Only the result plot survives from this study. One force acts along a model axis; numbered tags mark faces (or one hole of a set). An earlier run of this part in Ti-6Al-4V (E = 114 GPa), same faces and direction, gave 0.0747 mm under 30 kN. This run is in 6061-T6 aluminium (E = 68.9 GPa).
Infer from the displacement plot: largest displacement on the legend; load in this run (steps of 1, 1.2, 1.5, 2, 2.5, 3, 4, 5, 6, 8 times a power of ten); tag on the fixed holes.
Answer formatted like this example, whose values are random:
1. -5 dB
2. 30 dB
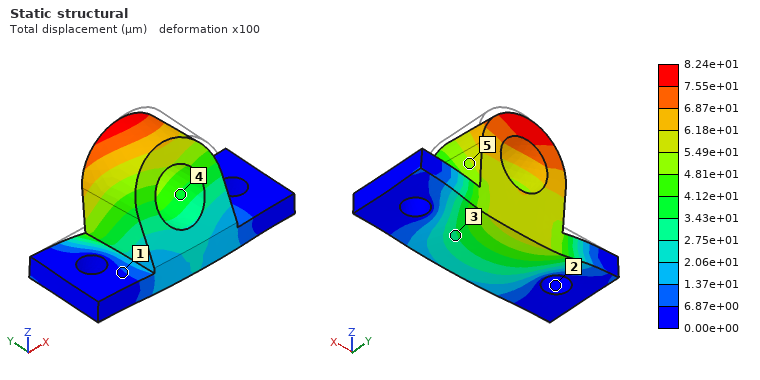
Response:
1. 8.24e+01 µm
2. 20 kN
3. 2
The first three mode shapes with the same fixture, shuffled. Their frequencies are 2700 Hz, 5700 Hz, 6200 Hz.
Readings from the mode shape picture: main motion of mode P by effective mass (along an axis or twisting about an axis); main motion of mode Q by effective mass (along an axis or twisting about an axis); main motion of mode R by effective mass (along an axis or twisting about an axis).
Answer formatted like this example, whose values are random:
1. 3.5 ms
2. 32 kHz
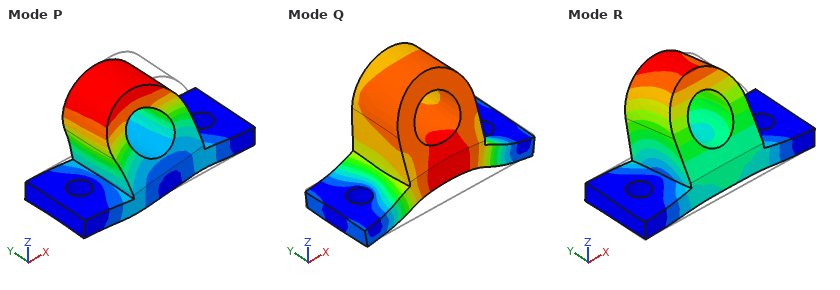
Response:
1. along X
2. along Z
3. along Y
